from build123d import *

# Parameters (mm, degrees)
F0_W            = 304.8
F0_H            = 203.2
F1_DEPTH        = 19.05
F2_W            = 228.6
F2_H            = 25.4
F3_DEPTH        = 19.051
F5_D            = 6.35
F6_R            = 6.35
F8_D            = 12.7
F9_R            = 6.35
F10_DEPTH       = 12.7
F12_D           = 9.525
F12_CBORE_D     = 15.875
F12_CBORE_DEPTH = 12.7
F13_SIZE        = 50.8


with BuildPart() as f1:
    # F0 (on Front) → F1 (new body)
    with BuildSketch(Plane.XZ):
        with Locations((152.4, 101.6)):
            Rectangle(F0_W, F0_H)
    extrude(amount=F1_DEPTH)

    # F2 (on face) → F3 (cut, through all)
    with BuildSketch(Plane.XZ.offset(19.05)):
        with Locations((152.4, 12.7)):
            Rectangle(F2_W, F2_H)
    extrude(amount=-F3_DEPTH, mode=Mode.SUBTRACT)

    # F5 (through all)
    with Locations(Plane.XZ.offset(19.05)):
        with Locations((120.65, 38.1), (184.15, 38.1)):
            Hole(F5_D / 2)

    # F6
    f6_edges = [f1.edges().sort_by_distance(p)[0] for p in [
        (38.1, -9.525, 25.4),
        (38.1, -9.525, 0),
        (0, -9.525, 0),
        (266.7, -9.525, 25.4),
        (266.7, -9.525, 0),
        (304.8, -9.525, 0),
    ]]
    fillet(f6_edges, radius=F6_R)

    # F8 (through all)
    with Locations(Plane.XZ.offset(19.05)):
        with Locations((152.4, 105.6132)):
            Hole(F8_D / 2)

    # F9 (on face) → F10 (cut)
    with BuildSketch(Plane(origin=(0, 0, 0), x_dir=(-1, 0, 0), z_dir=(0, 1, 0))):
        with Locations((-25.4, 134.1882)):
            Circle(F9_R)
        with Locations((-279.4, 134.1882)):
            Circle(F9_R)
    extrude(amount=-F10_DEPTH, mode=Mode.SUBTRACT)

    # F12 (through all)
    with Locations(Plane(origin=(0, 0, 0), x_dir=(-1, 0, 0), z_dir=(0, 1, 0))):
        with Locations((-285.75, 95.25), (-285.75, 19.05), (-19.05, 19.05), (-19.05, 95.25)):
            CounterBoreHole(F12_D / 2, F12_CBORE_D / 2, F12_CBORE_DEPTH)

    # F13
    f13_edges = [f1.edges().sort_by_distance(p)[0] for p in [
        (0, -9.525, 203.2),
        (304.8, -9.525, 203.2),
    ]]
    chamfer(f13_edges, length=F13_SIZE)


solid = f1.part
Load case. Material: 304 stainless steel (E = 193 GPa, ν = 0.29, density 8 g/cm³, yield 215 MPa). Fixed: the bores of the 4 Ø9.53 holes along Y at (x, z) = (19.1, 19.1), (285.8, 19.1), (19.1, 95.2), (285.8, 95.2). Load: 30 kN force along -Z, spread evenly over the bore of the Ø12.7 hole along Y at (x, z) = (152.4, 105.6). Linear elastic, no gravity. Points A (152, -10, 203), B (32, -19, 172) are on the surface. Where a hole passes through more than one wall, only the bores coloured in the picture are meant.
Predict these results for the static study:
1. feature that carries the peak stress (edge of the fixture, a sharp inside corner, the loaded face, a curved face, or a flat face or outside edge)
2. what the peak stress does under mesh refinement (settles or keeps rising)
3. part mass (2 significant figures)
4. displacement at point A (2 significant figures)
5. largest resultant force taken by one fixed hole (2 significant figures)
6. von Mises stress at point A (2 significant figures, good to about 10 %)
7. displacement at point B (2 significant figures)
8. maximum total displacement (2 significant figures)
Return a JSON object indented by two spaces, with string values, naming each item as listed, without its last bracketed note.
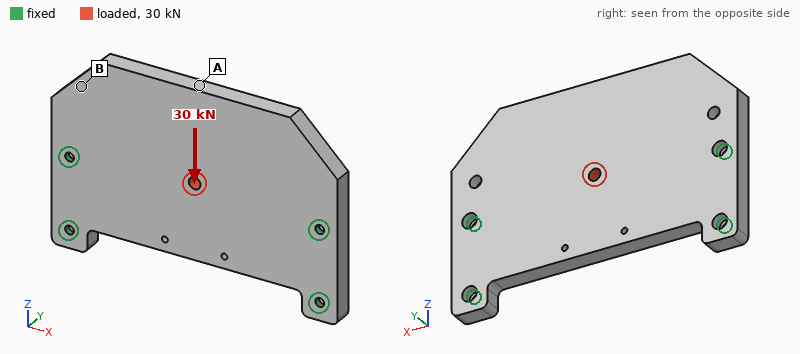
{
  "feature that carries the peak stress": "edge of the fixture",
  "what the peak stress does under mesh refinement": "keeps rising",
  "part mass": "8.0 kg",
  "displacement at point A": "20 µm",
  "largest resultant force taken by one fixed hole": "9.1 kN",
  "von Mises stress at point A": "17 MPa",
  "displacement at point B": "11 µm",
  "maximum total displacement": "21 µm"
}
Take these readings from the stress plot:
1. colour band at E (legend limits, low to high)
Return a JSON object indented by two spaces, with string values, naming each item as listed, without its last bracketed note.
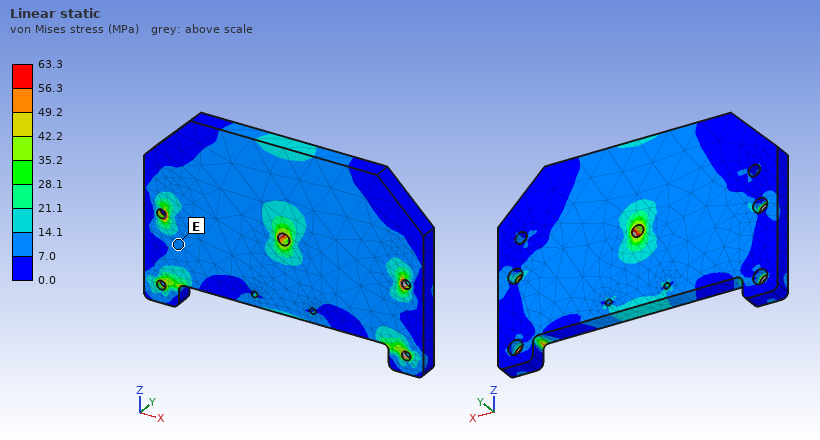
{
  "colour band at E": "7.0 to 14.1 MPa"
}
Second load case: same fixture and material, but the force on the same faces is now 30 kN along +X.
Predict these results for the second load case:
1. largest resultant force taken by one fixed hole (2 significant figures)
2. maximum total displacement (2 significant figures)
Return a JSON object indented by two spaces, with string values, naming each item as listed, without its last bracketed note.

{
  "largest resultant force taken by one fixed hole": "11 kN",
  "maximum total displacement": "13 µm"
}
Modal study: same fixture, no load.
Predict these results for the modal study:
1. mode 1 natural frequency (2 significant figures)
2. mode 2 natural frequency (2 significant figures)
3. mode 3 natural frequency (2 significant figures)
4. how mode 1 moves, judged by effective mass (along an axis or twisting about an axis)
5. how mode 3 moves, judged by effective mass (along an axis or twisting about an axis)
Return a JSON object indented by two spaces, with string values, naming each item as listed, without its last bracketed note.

{
  "mode 1 natural frequency": "620 Hz",
  "mode 2 natural frequency": "1200 Hz",
  "mode 3 natural frequency": "1500 Hz",
  "how mode 1 moves, judged by effective mass": "along Y",
  "how mode 3 moves, judged by effective mass": "twisting about Z"
}
